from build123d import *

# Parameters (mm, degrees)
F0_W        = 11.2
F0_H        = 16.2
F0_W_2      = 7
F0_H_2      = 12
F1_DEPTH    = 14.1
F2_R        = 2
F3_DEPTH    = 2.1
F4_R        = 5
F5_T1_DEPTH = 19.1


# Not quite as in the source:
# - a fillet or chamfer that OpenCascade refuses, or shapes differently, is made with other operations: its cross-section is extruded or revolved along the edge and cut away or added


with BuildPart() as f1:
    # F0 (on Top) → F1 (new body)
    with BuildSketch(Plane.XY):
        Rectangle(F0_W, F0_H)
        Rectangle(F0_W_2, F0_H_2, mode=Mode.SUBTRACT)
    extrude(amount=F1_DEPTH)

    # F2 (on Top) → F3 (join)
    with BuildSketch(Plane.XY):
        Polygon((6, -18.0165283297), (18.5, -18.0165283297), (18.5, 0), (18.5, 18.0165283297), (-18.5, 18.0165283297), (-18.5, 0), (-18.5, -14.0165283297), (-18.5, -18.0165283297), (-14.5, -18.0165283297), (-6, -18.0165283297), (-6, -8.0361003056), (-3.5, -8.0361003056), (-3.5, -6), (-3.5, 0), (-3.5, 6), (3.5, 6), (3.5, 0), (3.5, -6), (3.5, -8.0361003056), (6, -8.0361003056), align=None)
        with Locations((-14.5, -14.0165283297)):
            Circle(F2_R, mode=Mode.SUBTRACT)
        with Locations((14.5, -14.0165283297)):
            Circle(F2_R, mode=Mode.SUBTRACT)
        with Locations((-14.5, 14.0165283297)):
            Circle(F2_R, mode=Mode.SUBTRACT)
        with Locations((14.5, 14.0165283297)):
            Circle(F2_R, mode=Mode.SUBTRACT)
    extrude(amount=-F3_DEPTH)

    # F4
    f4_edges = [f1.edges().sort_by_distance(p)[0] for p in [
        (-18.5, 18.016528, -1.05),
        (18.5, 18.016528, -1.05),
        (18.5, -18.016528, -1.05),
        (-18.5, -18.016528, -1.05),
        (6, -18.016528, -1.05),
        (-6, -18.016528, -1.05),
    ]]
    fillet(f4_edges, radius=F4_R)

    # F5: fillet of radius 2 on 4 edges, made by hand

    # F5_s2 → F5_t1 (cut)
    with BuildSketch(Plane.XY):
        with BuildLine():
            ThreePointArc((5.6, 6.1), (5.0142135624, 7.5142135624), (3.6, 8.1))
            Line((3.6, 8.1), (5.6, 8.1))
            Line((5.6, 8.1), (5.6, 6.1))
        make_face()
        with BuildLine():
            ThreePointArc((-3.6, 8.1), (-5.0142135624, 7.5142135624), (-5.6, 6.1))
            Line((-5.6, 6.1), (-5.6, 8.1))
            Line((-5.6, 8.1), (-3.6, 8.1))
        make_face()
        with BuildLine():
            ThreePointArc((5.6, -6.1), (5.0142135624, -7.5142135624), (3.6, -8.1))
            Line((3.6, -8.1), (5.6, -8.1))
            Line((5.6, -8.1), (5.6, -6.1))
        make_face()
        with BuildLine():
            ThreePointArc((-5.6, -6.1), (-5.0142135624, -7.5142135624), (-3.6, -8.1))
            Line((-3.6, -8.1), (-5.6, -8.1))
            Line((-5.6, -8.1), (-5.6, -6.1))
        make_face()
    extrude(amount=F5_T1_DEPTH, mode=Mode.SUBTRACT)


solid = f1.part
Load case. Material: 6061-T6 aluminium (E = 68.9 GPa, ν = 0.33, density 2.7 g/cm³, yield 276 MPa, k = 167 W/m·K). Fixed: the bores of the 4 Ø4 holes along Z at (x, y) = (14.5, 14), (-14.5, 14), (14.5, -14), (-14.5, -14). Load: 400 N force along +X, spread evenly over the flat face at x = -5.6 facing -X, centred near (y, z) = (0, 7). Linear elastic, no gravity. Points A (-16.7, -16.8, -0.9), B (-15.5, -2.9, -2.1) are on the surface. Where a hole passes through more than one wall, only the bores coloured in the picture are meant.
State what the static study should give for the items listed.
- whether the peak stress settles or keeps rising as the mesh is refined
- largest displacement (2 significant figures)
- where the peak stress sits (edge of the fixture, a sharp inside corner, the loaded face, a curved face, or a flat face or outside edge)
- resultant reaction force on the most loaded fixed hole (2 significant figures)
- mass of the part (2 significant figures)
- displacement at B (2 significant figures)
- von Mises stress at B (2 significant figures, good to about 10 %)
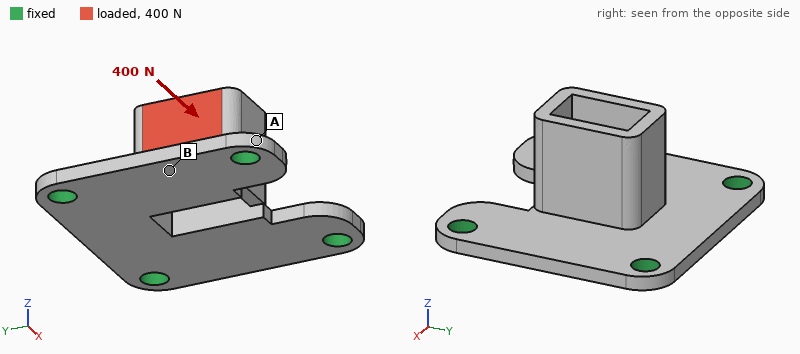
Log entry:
keeps rising
52 µm
a sharp inside corner
170 N
9.4 g
8.5 µm
15 MPa
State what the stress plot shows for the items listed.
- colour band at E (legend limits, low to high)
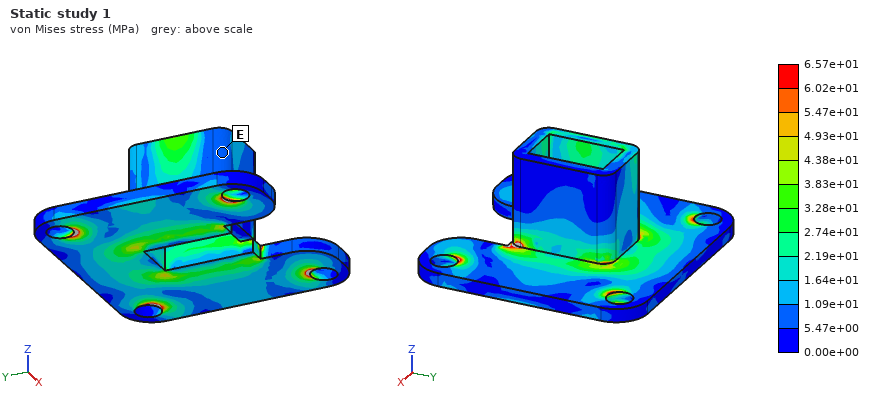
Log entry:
5.47e+00 to 1.09e+01 MPa
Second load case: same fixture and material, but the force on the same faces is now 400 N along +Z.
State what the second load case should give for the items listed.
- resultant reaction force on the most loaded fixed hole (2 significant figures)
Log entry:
180 N
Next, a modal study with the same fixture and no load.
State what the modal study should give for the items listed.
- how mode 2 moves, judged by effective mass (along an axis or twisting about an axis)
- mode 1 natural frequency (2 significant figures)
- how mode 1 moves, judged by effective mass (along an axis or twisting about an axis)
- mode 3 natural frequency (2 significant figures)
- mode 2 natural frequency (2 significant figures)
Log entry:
along X
7600 Hz
along Z
9200 Hz
8700 Hz
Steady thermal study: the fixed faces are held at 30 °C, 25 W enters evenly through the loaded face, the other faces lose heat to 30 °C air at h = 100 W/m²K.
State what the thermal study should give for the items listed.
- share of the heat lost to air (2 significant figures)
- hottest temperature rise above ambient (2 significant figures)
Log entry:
18 %
38 K
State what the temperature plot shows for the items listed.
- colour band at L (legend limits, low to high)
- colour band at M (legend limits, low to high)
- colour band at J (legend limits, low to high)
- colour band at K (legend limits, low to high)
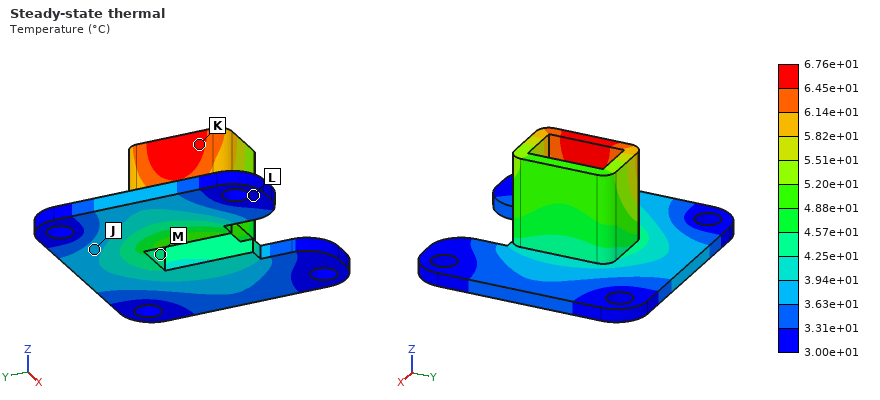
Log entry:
3.00e+01 to 3.31e+01 °C
4.25e+01 to 4.57e+01 °C
3.63e+01 to 3.94e+01 °C
6.45e+01 to 6.76e+01 °C
